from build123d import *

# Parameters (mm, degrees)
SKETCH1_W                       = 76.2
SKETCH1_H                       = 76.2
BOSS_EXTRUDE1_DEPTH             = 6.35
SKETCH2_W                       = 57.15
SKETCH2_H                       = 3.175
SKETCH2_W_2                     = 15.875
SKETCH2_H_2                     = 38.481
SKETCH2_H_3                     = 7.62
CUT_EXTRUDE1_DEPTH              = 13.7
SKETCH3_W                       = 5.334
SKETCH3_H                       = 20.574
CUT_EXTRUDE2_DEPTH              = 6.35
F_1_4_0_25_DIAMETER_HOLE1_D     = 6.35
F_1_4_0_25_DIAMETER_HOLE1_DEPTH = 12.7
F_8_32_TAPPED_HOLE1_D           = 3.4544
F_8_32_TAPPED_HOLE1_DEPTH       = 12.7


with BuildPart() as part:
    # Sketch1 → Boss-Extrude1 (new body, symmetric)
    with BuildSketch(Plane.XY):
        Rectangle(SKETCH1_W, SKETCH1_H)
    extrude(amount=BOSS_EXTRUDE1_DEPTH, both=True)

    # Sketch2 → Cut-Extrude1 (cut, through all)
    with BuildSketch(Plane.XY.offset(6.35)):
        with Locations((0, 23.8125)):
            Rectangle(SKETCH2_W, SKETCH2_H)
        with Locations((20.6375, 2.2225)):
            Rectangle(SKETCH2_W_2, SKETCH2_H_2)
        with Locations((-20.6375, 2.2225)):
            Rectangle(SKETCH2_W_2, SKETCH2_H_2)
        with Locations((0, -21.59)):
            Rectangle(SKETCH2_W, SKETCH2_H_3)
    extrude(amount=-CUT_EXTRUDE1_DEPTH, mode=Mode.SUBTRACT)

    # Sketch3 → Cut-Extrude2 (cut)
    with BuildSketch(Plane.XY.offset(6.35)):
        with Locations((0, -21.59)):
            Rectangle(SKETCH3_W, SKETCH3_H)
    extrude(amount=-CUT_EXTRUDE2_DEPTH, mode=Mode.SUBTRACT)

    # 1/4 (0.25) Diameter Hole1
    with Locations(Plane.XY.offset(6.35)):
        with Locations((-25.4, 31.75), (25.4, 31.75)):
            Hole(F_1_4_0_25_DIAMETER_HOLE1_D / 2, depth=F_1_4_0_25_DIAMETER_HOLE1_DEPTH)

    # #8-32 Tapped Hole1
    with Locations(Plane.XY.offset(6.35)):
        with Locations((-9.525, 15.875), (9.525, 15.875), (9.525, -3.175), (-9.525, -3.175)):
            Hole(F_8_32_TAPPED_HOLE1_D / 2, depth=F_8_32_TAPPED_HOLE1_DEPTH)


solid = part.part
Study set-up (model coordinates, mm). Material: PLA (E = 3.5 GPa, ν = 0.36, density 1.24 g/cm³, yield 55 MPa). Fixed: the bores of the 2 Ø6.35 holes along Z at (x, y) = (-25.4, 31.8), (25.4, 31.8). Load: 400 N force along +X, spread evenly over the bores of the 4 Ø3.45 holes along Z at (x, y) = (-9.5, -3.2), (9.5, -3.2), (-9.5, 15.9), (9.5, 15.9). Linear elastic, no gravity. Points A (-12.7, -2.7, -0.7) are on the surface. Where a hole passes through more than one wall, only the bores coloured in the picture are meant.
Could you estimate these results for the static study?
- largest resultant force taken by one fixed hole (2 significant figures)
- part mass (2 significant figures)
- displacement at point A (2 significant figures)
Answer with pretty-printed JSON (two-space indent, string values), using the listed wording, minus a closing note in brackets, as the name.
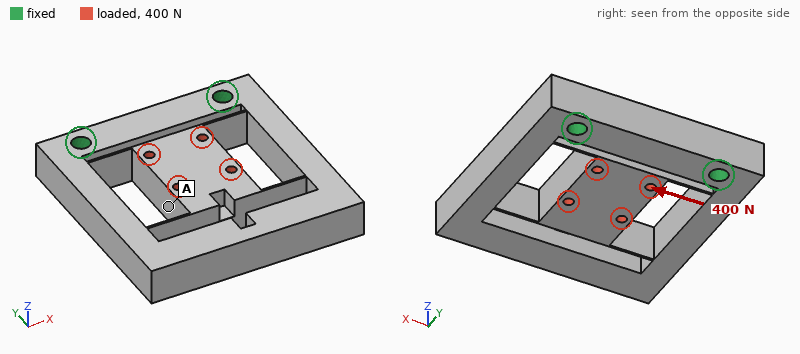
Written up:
{
  "largest resultant force taken by one fixed hole": "210 N",
  "part mass": "60 g",
  "displacement at point A": "0.43 mm"
}
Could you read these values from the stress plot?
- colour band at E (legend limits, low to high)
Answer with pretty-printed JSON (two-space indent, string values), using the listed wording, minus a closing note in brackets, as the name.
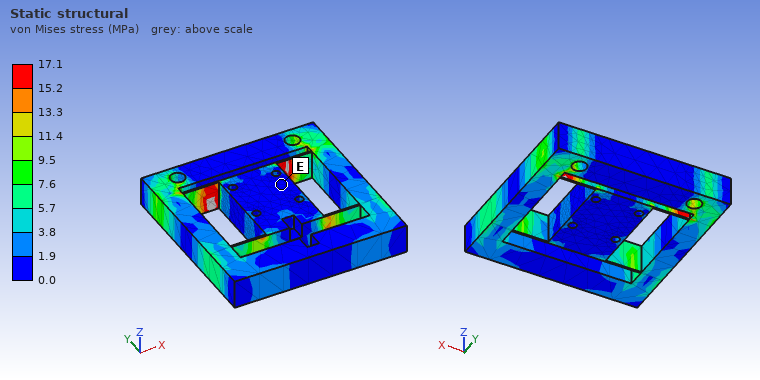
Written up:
{
  "colour band at E": "0.0 to 1.9 MPa"
}
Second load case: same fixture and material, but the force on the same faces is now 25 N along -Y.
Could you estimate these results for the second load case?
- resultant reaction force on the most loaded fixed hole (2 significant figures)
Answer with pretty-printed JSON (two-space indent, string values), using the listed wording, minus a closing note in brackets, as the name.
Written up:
{
  "resultant reaction force on the most loaded fixed hole": "13 N"
}
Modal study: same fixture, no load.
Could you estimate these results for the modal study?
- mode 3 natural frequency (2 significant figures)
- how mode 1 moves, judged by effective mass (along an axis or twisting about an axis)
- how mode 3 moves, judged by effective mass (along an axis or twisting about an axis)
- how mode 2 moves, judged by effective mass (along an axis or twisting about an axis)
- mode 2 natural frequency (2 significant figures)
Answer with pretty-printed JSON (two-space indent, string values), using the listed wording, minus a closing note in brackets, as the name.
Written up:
{
  "mode 3 natural frequency": "510 Hz",
  "how mode 1 moves, judged by effective mass": "along Y",
  "how mode 3 moves, judged by effective mass": "along X",
  "how mode 2 moves, judged by effective mass": "along Z",
  "mode 2 natural frequency": "370 Hz"
}
